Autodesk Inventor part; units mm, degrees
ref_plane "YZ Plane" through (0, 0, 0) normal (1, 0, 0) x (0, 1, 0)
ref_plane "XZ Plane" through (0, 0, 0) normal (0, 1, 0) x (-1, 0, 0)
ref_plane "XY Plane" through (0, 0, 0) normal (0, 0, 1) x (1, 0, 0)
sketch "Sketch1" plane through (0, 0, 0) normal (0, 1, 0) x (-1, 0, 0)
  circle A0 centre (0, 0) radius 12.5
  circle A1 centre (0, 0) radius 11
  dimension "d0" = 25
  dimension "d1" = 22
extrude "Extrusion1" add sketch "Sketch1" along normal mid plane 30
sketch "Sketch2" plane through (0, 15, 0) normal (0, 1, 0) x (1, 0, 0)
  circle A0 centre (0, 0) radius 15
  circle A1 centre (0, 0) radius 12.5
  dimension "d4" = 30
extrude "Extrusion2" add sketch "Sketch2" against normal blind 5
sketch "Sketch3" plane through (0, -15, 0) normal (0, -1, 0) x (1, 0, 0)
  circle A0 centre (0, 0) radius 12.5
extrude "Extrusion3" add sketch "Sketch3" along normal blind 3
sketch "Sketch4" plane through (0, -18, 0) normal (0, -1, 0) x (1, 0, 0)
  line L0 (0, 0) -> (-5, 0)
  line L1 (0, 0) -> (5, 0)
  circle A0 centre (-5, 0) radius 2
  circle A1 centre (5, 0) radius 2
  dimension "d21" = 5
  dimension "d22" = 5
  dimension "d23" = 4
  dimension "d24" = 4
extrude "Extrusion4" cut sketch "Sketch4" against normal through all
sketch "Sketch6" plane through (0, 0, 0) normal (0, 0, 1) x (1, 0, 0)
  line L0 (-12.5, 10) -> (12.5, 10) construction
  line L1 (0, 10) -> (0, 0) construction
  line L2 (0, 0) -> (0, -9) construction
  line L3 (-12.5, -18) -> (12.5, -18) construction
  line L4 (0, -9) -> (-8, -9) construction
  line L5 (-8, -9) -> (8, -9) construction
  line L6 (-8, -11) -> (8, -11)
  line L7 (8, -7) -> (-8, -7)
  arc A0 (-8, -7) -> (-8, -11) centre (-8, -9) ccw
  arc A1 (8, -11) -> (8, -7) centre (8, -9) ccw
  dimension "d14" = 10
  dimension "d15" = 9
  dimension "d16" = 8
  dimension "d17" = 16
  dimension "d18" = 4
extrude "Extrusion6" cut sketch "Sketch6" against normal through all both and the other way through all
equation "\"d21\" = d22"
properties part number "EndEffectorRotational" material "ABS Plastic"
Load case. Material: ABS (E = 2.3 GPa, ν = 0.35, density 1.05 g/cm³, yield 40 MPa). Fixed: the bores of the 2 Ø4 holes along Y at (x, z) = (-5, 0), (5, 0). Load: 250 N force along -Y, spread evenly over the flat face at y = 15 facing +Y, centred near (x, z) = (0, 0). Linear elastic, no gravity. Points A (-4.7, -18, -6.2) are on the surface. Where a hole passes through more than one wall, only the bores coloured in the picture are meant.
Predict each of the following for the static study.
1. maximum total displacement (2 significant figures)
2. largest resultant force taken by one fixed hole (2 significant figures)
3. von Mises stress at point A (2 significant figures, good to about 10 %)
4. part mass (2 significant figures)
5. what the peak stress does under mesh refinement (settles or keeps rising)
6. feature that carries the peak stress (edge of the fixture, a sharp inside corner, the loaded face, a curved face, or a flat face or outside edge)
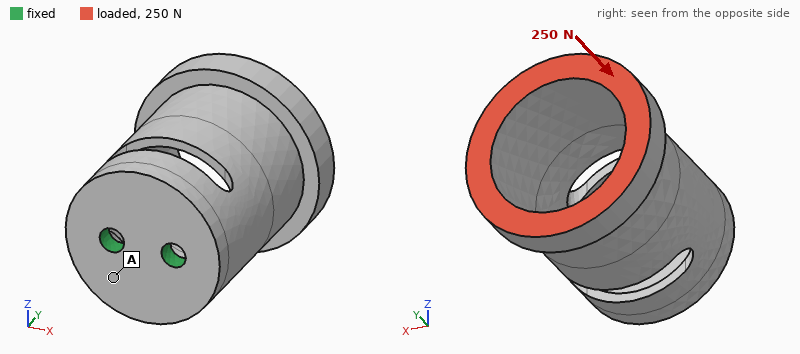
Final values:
0.20 mm
130 N
5.5 MPa
5.8 g
keeps rising
edge of the fixture
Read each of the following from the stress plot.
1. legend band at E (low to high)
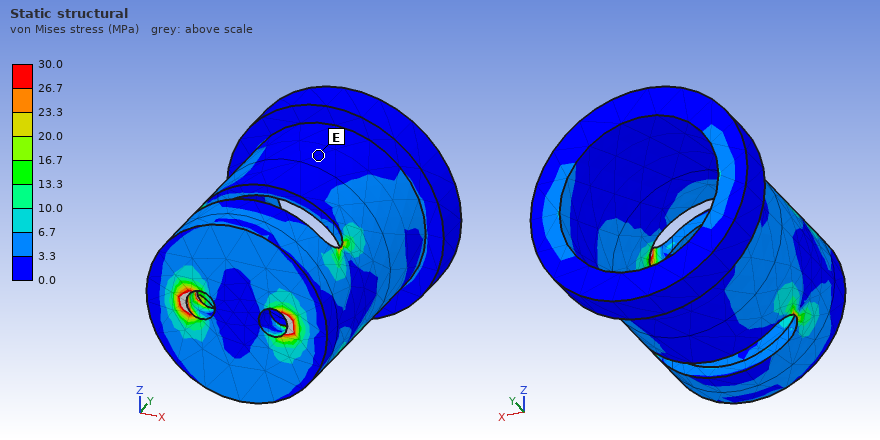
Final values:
0.0 to 3.3 MPa
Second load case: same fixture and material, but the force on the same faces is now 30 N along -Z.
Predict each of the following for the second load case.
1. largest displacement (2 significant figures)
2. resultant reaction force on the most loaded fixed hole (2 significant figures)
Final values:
0.56 mm
15 N
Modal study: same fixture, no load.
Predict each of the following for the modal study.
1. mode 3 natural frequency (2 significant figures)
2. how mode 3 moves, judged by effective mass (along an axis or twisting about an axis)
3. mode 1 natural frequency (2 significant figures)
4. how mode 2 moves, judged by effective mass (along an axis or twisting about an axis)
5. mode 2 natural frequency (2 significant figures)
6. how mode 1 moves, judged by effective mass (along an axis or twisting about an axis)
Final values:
2200 Hz
twisting about Y
800 Hz
along X
1100 Hz
along Z
